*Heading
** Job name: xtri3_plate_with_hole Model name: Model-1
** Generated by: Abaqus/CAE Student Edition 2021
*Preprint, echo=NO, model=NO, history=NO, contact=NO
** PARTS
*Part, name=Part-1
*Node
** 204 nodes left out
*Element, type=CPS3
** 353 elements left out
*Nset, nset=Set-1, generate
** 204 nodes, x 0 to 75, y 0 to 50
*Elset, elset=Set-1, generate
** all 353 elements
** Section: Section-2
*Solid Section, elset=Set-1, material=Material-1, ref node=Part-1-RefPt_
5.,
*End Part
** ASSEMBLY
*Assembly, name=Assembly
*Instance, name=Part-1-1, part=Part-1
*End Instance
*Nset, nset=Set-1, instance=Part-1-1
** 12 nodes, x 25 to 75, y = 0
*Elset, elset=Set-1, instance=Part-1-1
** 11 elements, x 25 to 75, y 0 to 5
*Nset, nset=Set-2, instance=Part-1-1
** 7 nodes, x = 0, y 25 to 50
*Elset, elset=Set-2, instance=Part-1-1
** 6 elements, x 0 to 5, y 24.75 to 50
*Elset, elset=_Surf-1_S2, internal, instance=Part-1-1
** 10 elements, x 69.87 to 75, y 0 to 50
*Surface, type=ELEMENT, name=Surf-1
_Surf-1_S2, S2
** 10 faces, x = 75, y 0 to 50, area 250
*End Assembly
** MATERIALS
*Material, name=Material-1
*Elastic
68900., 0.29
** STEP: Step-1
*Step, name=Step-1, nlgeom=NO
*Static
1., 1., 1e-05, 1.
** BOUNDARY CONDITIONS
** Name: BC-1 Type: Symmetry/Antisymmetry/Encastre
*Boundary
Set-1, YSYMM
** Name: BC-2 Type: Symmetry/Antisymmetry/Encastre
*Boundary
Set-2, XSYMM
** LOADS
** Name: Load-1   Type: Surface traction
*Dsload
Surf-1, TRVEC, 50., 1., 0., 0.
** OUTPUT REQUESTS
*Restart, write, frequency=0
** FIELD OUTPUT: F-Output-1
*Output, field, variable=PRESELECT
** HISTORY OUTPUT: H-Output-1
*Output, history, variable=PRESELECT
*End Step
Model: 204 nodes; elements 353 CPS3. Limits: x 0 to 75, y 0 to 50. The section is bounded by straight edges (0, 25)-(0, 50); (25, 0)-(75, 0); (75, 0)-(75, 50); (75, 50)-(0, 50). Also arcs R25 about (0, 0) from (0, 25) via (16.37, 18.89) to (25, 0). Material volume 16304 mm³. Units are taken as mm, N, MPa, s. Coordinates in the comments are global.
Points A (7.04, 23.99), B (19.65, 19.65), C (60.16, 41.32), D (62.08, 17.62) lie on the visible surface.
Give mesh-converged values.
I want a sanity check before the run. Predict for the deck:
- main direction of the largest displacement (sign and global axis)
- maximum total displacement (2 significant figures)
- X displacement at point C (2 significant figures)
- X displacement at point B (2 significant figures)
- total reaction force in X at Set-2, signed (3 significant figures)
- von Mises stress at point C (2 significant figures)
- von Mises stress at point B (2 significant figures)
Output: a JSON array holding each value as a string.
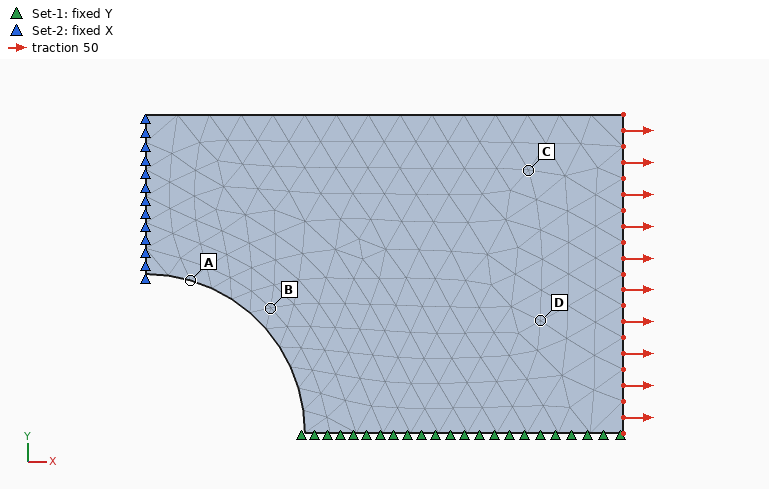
["+X", "0.10 mm", "0.063 mm", "0.053 mm", "-12500 N", "58 MPa", "60 MPa"]
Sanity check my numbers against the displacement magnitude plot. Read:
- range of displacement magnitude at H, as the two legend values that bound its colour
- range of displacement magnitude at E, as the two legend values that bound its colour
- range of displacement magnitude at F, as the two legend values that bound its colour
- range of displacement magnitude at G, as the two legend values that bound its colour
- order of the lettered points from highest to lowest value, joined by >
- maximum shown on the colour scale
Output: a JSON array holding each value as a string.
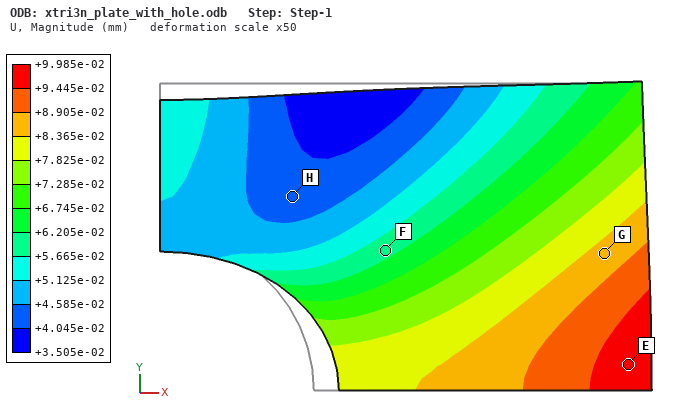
["+4.045e-02 to +4.585e-02 mm", "+9.445e-02 to +9.985e-02 mm", "+5.665e-02 to +6.205e-02 mm", "+8.365e-02 to +8.905e-02 mm", "E > G > F > H", "+9.985e-02 mm"]
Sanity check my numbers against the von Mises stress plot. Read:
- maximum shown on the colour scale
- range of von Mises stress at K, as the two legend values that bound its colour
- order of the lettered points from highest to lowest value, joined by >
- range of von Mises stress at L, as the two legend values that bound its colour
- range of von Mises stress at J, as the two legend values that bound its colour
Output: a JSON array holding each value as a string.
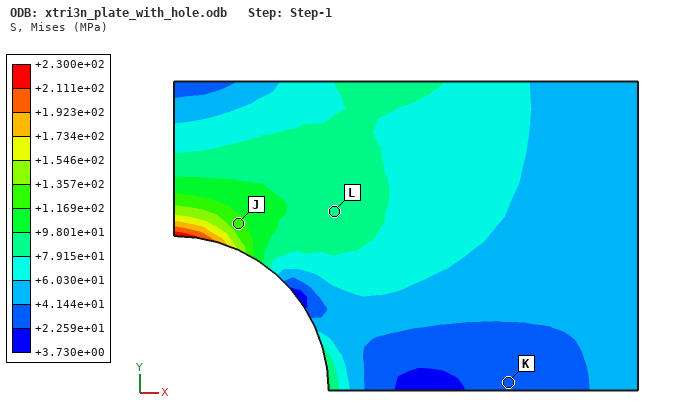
["+2.300e+02 MPa", "+2.259e+01 to +4.144e+01 MPa", "J > L > K", "+7.915e+01 to +9.801e+01 MPa", "+1.169e+02 to +1.357e+02 MPa"]
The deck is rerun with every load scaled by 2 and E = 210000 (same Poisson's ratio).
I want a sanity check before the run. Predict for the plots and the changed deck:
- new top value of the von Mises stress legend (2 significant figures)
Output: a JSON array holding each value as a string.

["460 MPa"]
